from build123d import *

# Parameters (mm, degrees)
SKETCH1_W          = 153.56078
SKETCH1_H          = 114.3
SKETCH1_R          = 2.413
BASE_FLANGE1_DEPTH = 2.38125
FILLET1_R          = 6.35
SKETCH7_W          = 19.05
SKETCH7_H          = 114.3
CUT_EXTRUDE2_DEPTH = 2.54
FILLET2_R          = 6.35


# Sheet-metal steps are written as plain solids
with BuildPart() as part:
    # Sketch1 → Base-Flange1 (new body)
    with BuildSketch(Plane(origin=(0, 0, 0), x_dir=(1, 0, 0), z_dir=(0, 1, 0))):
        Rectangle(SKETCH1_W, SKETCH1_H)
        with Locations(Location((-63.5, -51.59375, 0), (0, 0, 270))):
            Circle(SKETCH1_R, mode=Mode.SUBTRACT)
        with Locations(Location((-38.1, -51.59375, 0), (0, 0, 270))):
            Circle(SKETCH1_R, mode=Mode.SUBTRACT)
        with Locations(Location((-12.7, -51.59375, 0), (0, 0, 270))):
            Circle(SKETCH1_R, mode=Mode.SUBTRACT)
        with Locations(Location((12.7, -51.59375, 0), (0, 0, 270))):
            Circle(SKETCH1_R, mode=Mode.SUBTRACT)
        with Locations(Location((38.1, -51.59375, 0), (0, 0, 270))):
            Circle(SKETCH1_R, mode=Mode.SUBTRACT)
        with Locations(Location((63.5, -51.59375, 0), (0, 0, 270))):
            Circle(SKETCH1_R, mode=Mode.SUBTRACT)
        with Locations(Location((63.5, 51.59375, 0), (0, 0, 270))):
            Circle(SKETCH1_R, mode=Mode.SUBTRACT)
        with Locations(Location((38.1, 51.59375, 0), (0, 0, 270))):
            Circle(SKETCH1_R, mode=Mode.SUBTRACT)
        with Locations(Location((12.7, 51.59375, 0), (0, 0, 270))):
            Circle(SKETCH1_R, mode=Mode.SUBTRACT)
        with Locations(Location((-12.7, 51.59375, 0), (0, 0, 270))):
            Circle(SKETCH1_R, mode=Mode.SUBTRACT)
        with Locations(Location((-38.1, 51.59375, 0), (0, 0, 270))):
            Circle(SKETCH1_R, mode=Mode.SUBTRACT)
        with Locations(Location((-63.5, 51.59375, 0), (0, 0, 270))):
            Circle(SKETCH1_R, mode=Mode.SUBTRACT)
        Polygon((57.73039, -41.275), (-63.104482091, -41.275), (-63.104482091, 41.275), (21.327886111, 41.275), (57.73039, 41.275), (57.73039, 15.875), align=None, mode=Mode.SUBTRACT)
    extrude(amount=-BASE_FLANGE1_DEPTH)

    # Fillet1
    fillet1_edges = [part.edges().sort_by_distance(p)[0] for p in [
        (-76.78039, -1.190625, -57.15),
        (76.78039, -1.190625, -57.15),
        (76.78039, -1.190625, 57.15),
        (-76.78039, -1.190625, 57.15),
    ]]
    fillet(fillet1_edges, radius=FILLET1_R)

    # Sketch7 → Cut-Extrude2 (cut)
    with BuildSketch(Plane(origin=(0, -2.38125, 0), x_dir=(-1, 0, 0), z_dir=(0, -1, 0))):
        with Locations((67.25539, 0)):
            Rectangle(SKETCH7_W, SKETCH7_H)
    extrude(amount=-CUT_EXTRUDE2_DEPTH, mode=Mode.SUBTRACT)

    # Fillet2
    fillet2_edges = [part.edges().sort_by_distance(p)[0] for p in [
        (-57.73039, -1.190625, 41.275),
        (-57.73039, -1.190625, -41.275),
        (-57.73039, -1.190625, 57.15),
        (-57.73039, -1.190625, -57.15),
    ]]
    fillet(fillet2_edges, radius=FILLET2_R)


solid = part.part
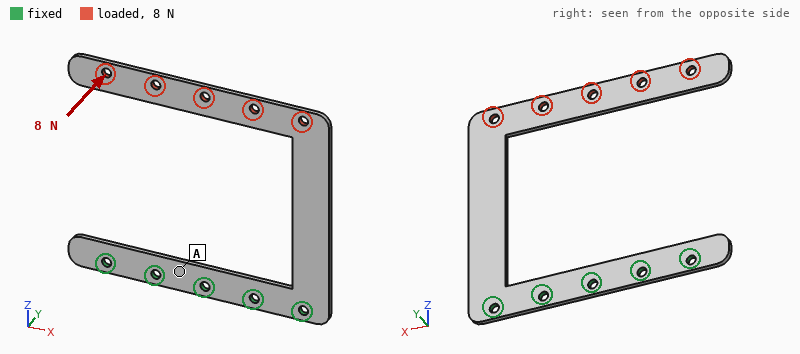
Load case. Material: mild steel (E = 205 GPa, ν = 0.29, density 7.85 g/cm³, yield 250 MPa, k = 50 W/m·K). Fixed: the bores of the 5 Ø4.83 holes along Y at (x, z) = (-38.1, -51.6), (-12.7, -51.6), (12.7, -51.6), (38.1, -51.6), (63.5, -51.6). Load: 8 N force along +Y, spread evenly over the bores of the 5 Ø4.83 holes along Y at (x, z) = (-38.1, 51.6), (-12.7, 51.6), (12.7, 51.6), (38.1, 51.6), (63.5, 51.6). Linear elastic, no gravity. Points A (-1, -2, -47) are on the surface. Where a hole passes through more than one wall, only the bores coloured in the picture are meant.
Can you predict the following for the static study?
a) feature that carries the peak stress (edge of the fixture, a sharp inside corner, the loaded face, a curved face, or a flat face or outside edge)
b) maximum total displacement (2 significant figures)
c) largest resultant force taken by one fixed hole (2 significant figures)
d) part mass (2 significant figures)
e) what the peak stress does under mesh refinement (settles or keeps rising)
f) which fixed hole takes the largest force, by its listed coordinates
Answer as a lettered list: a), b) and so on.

a) edge of the fixture
b) 1.8 mm
c) 6.1 N
d) 100 g
e) keeps rising
f) (63.5, -51.6)
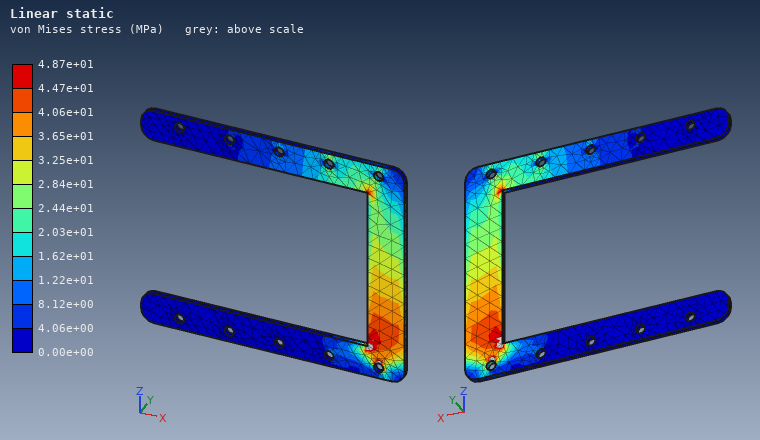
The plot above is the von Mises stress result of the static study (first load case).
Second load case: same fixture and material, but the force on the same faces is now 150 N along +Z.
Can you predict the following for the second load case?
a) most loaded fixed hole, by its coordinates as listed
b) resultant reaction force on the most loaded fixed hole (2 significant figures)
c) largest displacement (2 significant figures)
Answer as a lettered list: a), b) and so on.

a) (38.1, -51.6)
b) 290 N
c) 0.59 mm
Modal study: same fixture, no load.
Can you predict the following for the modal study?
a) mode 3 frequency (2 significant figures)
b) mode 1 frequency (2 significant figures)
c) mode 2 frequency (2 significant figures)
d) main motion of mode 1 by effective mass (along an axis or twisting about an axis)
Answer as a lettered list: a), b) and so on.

a) 430 Hz
b) 64 Hz
c) 160 Hz
d) along Y
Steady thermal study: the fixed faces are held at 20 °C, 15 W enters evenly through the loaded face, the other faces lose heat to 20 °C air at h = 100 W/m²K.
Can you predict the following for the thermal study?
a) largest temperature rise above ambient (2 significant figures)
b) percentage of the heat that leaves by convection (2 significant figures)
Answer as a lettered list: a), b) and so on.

a) 38 K
b) 100 %
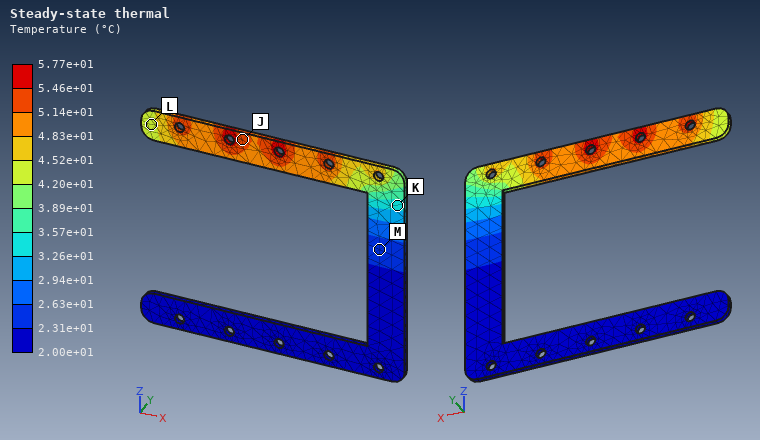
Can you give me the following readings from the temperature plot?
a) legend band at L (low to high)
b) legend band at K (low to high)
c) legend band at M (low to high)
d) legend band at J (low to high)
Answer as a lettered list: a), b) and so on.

a) 4.20e+01 to 4.52e+01 °C
b) 3.26e+01 to 3.57e+01 °C
c) 2.31e+01 to 2.63e+01 °C
d) 5.14e+01 to 5.46e+01 °C
